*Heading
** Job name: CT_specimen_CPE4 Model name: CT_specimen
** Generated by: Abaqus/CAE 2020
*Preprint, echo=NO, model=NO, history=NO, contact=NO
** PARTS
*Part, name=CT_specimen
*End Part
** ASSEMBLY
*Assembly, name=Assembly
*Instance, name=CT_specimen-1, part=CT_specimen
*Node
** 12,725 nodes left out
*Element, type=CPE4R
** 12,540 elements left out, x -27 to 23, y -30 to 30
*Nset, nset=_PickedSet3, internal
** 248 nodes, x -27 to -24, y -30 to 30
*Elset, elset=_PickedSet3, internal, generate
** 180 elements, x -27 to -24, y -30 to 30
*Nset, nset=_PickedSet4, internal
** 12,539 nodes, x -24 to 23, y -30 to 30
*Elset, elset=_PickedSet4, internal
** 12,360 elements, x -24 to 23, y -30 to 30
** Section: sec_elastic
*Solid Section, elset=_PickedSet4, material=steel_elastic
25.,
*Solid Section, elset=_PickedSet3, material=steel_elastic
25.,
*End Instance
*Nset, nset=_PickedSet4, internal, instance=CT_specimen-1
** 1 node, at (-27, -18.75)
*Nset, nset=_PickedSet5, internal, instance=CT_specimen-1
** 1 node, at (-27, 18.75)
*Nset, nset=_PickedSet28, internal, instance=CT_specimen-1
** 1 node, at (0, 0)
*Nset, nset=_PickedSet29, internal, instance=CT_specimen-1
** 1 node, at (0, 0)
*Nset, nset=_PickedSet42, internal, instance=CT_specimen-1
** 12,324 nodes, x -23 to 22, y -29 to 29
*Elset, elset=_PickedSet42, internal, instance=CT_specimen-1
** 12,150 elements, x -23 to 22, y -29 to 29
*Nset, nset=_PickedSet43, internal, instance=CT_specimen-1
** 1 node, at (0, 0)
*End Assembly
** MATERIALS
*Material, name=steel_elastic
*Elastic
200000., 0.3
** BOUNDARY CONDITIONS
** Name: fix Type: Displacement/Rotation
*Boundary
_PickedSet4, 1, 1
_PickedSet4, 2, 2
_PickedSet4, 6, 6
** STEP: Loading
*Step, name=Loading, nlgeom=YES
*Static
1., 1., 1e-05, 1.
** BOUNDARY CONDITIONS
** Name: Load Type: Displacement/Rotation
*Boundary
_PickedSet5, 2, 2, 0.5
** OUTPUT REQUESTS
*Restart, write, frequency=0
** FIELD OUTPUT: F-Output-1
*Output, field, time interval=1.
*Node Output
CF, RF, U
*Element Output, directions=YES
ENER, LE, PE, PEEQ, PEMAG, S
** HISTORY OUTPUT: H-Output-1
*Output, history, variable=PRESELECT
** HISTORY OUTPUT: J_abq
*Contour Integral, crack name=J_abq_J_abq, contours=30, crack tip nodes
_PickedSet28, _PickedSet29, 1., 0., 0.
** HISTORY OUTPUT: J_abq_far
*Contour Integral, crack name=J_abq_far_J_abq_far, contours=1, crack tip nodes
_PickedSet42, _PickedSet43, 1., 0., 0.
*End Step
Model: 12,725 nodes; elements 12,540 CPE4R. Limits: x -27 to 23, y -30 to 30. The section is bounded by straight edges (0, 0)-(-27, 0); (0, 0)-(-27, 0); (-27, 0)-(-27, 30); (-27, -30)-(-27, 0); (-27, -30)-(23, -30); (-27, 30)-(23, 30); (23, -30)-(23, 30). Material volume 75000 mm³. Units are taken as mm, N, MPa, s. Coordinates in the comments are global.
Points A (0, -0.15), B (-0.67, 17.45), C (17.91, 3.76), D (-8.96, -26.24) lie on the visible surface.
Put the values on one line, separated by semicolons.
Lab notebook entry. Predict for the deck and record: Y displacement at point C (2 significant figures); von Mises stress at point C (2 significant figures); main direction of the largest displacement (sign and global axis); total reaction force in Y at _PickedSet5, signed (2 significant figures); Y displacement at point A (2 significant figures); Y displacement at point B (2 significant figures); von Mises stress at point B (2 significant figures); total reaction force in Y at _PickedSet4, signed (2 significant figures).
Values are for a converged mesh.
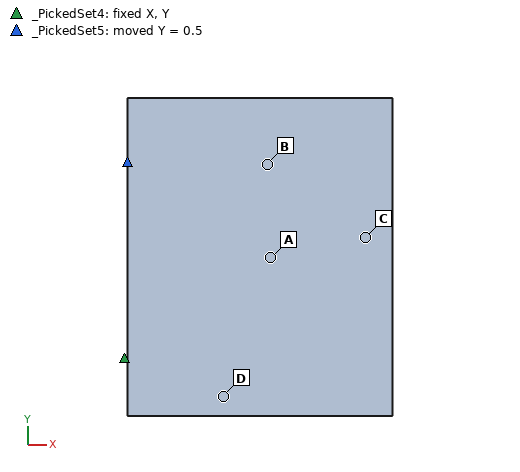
0.24 mm; 350 MPa; +Y; 56000 N; 0.25 mm; 0.29 mm; 180 MPa; -56000 N
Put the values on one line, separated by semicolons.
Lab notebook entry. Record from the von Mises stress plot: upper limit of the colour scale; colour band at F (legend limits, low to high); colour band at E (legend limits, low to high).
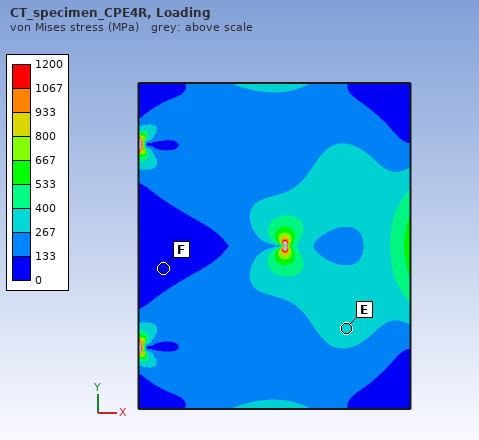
1200 MPa; 0 to 133 MPa; 267 to 400 MPa
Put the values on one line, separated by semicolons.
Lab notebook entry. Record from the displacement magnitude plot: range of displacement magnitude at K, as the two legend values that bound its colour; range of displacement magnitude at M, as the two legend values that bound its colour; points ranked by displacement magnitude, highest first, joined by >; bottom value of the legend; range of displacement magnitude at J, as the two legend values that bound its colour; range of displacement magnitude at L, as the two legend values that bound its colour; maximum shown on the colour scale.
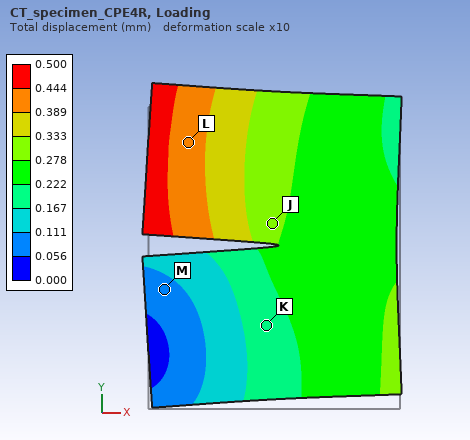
0.167 to 0.222 mm; 0.056 to 0.111 mm; L > J > K > M; 0.000 mm; 0.278 to 0.333 mm; 0.389 to 0.444 mm; 0.500 mm
